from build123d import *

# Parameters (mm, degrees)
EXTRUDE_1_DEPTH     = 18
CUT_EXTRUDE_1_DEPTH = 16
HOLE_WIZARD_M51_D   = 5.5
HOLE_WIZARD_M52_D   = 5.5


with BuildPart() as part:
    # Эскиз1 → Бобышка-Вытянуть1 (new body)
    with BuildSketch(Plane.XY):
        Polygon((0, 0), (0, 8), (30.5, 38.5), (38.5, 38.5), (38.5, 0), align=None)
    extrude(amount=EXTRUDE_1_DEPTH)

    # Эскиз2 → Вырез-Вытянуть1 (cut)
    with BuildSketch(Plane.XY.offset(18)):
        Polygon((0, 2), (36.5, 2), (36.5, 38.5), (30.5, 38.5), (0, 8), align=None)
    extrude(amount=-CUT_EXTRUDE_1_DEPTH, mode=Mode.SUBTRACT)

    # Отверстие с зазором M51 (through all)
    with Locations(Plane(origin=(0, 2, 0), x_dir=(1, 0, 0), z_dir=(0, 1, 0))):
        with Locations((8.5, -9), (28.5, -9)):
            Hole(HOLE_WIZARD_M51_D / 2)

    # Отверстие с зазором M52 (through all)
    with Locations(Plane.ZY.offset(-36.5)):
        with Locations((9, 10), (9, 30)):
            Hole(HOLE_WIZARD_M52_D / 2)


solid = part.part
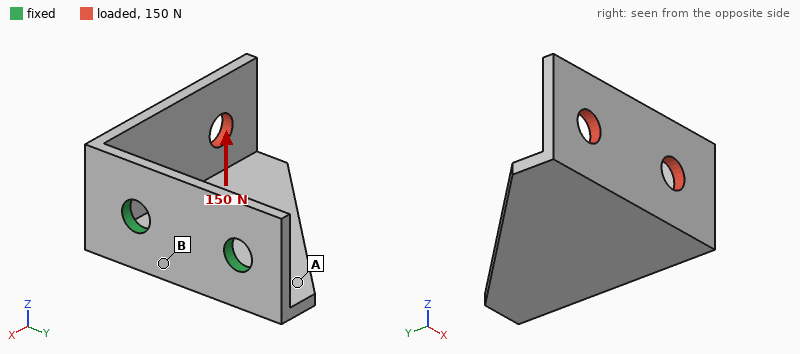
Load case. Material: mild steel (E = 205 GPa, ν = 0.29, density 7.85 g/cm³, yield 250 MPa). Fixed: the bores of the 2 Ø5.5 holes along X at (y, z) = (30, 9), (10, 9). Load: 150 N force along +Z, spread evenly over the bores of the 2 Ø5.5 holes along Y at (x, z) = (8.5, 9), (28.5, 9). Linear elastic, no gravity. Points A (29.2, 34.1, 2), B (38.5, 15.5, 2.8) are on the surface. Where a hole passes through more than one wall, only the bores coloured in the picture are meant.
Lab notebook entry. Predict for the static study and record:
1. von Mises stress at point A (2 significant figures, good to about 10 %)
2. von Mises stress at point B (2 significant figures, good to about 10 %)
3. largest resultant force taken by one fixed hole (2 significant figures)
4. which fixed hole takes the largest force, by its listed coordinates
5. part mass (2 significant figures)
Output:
21 MPa
43 MPa
180 N
(10, 9)
33 g
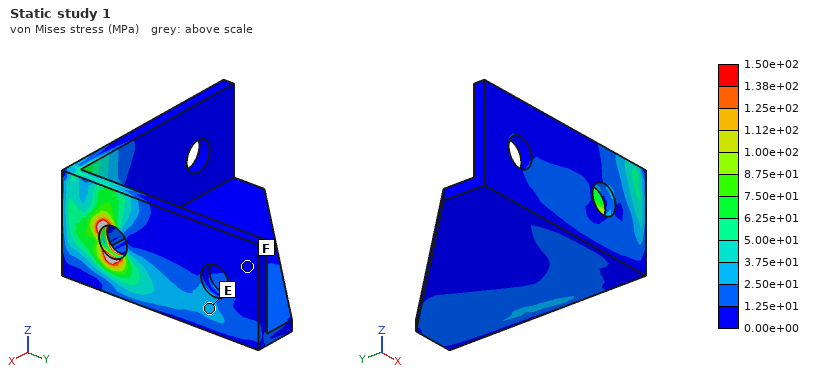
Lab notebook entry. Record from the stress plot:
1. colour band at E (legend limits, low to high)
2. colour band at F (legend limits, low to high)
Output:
2.50e+01 to 3.75e+01 MPa
0.00e+00 to 1.25e+01 MPa
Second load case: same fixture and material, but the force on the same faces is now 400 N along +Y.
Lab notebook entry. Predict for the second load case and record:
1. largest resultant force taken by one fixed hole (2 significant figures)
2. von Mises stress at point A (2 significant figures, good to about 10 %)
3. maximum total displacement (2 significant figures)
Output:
390 N
21 MPa
0.16 mm
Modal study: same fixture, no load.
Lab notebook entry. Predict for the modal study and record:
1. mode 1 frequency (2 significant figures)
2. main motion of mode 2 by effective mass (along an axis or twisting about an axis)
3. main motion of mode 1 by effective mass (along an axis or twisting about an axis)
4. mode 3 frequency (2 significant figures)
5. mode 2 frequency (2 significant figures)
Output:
1900 Hz
along Y
along Z
6400 Hz
3000 Hz
